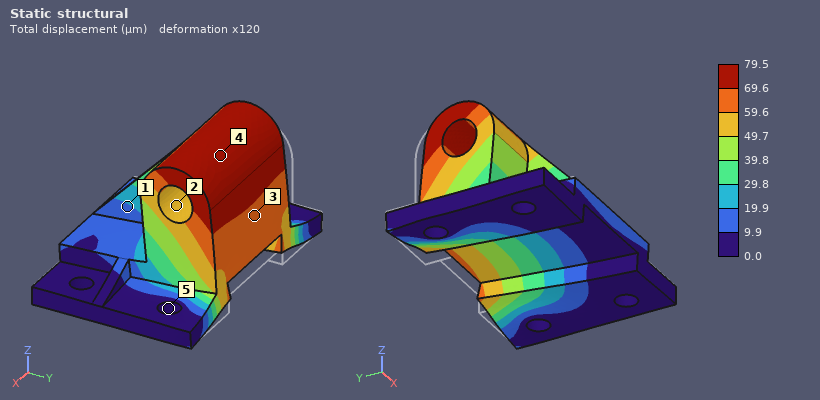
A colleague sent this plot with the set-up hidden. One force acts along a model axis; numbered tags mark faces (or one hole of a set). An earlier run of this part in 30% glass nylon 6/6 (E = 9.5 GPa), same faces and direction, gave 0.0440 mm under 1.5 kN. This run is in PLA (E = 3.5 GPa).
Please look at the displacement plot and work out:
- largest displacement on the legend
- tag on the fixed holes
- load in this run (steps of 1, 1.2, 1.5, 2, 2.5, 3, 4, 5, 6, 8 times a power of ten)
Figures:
79.5 µm
5
1 kN
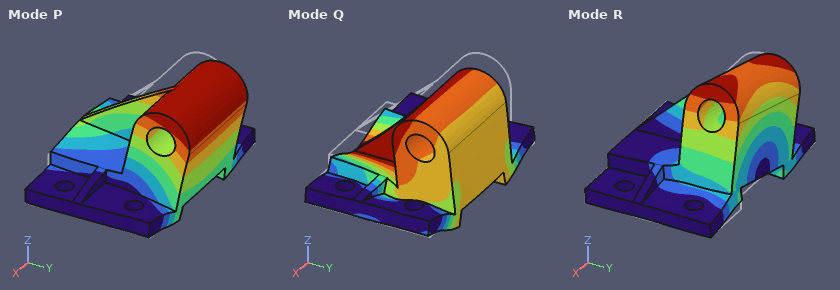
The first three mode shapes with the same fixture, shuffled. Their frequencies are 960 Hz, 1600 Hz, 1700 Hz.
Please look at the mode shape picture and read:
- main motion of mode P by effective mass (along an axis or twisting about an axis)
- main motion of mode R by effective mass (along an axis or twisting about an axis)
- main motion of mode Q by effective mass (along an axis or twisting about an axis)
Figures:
along Y
along X
along Z
